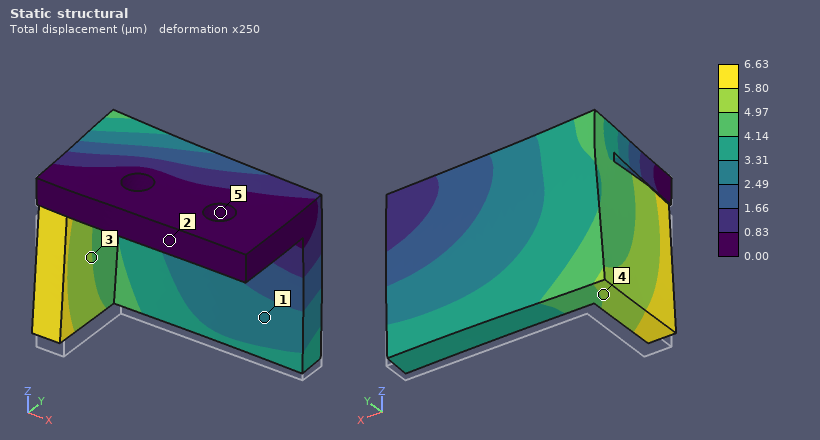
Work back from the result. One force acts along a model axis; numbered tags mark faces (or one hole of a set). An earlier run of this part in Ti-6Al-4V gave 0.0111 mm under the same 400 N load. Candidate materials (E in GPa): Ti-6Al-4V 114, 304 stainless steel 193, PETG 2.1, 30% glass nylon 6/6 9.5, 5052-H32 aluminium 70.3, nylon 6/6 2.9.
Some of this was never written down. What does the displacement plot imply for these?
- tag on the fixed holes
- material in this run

5
304 stainless steel
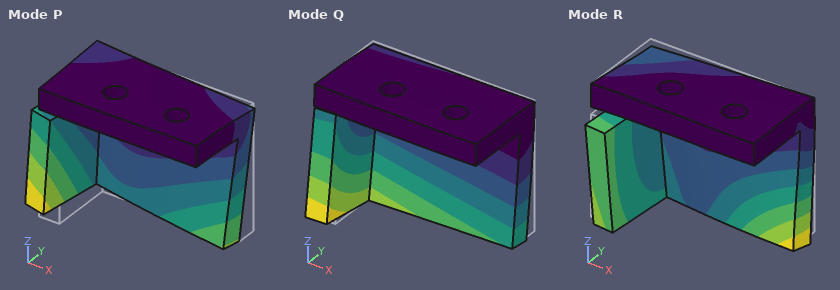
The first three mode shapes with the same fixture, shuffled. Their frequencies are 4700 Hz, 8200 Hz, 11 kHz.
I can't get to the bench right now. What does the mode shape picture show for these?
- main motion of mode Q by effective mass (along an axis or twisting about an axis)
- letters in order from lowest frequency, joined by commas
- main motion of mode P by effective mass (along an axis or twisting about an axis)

along Y
Q, P, R
along X
